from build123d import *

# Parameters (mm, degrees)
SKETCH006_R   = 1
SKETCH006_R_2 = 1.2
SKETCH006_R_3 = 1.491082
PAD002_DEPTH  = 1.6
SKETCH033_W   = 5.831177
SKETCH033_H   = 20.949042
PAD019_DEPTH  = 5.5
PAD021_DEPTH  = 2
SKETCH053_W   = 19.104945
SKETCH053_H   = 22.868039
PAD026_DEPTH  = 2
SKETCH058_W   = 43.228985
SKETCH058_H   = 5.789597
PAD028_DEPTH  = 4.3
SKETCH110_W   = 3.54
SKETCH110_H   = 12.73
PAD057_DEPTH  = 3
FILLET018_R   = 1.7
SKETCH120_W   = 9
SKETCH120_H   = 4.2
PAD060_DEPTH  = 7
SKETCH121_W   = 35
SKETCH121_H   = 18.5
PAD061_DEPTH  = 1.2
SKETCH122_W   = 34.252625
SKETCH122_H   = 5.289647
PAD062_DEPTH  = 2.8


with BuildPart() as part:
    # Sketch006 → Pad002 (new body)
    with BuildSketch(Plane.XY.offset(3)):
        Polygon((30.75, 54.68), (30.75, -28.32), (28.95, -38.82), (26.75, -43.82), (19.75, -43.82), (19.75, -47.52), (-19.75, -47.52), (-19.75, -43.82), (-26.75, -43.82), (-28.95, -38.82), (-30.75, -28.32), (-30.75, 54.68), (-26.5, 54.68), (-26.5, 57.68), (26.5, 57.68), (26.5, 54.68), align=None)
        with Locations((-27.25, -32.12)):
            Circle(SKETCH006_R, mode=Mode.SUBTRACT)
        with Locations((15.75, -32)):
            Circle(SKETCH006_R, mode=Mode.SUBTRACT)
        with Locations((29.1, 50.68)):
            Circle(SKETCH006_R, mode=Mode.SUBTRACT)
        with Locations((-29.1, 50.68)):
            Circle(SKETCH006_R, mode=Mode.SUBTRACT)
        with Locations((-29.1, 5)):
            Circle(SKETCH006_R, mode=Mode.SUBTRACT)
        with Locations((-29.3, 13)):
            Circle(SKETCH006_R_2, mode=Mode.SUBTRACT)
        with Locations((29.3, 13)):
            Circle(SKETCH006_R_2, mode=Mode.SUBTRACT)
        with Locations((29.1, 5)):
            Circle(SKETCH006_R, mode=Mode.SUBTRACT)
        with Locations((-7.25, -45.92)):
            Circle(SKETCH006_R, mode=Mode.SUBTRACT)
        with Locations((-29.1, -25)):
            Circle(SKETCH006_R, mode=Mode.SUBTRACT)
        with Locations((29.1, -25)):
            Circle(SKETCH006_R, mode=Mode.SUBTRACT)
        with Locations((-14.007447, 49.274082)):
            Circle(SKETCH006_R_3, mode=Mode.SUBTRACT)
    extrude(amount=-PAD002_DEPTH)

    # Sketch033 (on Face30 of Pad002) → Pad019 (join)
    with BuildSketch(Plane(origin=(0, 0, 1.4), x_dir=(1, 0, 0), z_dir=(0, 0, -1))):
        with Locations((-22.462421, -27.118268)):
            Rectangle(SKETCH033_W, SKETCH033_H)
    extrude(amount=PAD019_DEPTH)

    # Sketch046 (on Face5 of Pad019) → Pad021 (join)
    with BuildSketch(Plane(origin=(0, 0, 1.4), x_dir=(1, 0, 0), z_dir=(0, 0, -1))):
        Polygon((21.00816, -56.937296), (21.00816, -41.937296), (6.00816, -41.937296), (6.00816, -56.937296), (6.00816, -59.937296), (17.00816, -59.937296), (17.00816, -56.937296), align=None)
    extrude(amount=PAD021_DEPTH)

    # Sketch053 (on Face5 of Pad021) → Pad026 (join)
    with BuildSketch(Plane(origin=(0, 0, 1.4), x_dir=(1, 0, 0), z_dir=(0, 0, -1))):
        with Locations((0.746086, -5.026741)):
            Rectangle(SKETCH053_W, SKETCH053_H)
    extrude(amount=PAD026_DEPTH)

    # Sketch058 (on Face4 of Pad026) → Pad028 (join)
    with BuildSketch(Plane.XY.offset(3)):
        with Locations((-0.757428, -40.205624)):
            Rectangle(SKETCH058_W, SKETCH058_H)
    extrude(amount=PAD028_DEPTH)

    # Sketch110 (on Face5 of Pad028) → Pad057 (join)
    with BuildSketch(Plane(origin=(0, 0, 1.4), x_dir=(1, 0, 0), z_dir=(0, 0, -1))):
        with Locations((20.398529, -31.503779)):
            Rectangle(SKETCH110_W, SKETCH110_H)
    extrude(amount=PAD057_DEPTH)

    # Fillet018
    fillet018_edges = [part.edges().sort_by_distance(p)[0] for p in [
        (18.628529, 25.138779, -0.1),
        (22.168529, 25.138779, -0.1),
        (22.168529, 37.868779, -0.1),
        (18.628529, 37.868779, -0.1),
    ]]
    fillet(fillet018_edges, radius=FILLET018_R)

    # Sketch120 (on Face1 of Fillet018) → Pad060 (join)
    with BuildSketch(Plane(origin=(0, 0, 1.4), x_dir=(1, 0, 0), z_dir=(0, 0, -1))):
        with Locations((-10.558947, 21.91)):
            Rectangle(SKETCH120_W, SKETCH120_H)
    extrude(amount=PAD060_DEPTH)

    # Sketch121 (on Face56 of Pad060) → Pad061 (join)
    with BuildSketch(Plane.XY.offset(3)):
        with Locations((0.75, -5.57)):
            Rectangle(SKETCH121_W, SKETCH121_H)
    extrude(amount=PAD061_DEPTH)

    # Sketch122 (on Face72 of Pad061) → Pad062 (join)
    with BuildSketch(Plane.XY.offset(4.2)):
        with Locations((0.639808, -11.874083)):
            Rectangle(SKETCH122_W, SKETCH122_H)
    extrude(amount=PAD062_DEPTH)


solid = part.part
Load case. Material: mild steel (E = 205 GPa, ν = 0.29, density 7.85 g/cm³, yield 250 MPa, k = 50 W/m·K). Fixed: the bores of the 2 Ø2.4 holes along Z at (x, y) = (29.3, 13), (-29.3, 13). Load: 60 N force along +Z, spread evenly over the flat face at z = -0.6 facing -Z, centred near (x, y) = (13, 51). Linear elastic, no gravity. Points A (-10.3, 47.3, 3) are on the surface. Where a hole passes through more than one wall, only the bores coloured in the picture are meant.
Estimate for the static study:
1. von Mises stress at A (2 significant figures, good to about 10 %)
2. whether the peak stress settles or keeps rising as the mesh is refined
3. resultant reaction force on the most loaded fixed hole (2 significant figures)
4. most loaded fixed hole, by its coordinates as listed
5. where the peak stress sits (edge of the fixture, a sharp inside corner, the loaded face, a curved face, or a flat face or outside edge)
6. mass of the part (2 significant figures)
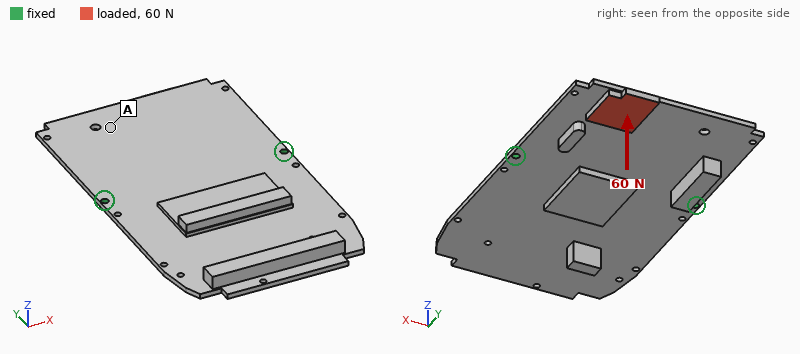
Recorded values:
28 MPa
keeps rising
49 N
(29.3, 13)
edge of the fixture
120 g
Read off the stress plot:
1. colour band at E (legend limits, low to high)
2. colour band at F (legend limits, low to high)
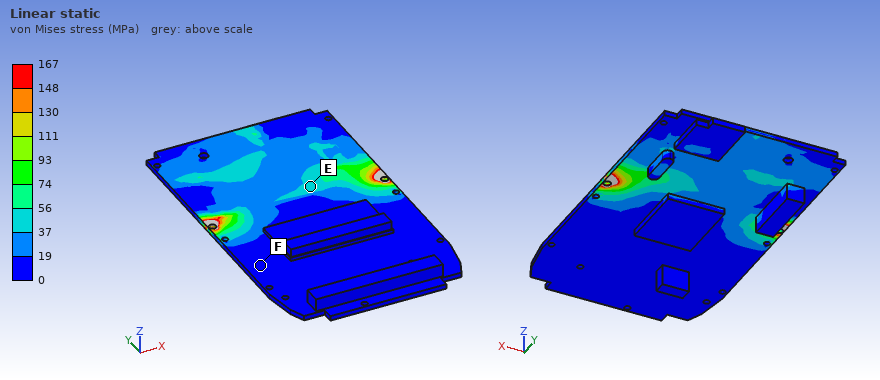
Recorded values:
37 to 56 MPa
0 to 19 MPa
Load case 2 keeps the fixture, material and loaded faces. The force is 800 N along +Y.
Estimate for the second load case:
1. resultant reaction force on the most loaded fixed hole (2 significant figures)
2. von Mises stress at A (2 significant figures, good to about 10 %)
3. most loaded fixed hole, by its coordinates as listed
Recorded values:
580 N
58 MPa
(29.3, 13)
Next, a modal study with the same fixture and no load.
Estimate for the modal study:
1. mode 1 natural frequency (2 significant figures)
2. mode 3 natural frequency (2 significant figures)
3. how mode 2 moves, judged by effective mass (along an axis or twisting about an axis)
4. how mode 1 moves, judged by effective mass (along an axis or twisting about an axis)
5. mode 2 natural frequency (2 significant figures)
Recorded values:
270 Hz
1400 Hz
along Z
along Z
650 Hz
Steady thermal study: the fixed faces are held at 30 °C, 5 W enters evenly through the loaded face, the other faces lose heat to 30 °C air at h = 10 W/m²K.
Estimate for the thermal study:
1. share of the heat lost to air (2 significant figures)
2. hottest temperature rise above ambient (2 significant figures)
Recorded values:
41 %
49 K
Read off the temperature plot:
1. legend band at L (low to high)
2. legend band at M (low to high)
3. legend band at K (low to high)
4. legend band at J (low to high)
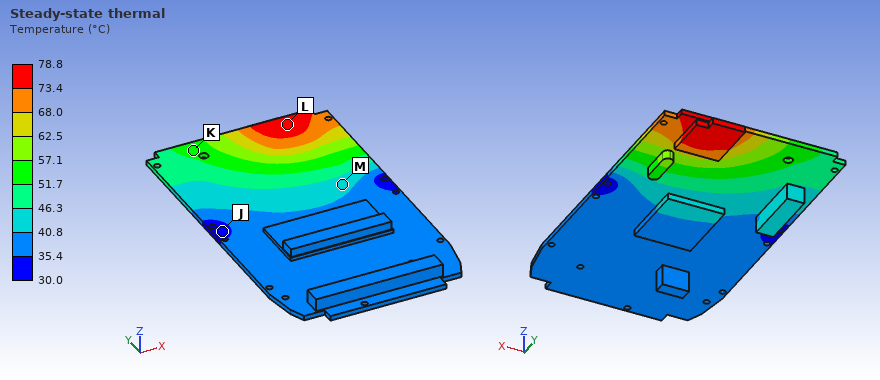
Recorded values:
73.4 to 78.8 °C
40.8 to 46.3 °C
51.7 to 57.1 °C
30.0 to 35.4 °C
